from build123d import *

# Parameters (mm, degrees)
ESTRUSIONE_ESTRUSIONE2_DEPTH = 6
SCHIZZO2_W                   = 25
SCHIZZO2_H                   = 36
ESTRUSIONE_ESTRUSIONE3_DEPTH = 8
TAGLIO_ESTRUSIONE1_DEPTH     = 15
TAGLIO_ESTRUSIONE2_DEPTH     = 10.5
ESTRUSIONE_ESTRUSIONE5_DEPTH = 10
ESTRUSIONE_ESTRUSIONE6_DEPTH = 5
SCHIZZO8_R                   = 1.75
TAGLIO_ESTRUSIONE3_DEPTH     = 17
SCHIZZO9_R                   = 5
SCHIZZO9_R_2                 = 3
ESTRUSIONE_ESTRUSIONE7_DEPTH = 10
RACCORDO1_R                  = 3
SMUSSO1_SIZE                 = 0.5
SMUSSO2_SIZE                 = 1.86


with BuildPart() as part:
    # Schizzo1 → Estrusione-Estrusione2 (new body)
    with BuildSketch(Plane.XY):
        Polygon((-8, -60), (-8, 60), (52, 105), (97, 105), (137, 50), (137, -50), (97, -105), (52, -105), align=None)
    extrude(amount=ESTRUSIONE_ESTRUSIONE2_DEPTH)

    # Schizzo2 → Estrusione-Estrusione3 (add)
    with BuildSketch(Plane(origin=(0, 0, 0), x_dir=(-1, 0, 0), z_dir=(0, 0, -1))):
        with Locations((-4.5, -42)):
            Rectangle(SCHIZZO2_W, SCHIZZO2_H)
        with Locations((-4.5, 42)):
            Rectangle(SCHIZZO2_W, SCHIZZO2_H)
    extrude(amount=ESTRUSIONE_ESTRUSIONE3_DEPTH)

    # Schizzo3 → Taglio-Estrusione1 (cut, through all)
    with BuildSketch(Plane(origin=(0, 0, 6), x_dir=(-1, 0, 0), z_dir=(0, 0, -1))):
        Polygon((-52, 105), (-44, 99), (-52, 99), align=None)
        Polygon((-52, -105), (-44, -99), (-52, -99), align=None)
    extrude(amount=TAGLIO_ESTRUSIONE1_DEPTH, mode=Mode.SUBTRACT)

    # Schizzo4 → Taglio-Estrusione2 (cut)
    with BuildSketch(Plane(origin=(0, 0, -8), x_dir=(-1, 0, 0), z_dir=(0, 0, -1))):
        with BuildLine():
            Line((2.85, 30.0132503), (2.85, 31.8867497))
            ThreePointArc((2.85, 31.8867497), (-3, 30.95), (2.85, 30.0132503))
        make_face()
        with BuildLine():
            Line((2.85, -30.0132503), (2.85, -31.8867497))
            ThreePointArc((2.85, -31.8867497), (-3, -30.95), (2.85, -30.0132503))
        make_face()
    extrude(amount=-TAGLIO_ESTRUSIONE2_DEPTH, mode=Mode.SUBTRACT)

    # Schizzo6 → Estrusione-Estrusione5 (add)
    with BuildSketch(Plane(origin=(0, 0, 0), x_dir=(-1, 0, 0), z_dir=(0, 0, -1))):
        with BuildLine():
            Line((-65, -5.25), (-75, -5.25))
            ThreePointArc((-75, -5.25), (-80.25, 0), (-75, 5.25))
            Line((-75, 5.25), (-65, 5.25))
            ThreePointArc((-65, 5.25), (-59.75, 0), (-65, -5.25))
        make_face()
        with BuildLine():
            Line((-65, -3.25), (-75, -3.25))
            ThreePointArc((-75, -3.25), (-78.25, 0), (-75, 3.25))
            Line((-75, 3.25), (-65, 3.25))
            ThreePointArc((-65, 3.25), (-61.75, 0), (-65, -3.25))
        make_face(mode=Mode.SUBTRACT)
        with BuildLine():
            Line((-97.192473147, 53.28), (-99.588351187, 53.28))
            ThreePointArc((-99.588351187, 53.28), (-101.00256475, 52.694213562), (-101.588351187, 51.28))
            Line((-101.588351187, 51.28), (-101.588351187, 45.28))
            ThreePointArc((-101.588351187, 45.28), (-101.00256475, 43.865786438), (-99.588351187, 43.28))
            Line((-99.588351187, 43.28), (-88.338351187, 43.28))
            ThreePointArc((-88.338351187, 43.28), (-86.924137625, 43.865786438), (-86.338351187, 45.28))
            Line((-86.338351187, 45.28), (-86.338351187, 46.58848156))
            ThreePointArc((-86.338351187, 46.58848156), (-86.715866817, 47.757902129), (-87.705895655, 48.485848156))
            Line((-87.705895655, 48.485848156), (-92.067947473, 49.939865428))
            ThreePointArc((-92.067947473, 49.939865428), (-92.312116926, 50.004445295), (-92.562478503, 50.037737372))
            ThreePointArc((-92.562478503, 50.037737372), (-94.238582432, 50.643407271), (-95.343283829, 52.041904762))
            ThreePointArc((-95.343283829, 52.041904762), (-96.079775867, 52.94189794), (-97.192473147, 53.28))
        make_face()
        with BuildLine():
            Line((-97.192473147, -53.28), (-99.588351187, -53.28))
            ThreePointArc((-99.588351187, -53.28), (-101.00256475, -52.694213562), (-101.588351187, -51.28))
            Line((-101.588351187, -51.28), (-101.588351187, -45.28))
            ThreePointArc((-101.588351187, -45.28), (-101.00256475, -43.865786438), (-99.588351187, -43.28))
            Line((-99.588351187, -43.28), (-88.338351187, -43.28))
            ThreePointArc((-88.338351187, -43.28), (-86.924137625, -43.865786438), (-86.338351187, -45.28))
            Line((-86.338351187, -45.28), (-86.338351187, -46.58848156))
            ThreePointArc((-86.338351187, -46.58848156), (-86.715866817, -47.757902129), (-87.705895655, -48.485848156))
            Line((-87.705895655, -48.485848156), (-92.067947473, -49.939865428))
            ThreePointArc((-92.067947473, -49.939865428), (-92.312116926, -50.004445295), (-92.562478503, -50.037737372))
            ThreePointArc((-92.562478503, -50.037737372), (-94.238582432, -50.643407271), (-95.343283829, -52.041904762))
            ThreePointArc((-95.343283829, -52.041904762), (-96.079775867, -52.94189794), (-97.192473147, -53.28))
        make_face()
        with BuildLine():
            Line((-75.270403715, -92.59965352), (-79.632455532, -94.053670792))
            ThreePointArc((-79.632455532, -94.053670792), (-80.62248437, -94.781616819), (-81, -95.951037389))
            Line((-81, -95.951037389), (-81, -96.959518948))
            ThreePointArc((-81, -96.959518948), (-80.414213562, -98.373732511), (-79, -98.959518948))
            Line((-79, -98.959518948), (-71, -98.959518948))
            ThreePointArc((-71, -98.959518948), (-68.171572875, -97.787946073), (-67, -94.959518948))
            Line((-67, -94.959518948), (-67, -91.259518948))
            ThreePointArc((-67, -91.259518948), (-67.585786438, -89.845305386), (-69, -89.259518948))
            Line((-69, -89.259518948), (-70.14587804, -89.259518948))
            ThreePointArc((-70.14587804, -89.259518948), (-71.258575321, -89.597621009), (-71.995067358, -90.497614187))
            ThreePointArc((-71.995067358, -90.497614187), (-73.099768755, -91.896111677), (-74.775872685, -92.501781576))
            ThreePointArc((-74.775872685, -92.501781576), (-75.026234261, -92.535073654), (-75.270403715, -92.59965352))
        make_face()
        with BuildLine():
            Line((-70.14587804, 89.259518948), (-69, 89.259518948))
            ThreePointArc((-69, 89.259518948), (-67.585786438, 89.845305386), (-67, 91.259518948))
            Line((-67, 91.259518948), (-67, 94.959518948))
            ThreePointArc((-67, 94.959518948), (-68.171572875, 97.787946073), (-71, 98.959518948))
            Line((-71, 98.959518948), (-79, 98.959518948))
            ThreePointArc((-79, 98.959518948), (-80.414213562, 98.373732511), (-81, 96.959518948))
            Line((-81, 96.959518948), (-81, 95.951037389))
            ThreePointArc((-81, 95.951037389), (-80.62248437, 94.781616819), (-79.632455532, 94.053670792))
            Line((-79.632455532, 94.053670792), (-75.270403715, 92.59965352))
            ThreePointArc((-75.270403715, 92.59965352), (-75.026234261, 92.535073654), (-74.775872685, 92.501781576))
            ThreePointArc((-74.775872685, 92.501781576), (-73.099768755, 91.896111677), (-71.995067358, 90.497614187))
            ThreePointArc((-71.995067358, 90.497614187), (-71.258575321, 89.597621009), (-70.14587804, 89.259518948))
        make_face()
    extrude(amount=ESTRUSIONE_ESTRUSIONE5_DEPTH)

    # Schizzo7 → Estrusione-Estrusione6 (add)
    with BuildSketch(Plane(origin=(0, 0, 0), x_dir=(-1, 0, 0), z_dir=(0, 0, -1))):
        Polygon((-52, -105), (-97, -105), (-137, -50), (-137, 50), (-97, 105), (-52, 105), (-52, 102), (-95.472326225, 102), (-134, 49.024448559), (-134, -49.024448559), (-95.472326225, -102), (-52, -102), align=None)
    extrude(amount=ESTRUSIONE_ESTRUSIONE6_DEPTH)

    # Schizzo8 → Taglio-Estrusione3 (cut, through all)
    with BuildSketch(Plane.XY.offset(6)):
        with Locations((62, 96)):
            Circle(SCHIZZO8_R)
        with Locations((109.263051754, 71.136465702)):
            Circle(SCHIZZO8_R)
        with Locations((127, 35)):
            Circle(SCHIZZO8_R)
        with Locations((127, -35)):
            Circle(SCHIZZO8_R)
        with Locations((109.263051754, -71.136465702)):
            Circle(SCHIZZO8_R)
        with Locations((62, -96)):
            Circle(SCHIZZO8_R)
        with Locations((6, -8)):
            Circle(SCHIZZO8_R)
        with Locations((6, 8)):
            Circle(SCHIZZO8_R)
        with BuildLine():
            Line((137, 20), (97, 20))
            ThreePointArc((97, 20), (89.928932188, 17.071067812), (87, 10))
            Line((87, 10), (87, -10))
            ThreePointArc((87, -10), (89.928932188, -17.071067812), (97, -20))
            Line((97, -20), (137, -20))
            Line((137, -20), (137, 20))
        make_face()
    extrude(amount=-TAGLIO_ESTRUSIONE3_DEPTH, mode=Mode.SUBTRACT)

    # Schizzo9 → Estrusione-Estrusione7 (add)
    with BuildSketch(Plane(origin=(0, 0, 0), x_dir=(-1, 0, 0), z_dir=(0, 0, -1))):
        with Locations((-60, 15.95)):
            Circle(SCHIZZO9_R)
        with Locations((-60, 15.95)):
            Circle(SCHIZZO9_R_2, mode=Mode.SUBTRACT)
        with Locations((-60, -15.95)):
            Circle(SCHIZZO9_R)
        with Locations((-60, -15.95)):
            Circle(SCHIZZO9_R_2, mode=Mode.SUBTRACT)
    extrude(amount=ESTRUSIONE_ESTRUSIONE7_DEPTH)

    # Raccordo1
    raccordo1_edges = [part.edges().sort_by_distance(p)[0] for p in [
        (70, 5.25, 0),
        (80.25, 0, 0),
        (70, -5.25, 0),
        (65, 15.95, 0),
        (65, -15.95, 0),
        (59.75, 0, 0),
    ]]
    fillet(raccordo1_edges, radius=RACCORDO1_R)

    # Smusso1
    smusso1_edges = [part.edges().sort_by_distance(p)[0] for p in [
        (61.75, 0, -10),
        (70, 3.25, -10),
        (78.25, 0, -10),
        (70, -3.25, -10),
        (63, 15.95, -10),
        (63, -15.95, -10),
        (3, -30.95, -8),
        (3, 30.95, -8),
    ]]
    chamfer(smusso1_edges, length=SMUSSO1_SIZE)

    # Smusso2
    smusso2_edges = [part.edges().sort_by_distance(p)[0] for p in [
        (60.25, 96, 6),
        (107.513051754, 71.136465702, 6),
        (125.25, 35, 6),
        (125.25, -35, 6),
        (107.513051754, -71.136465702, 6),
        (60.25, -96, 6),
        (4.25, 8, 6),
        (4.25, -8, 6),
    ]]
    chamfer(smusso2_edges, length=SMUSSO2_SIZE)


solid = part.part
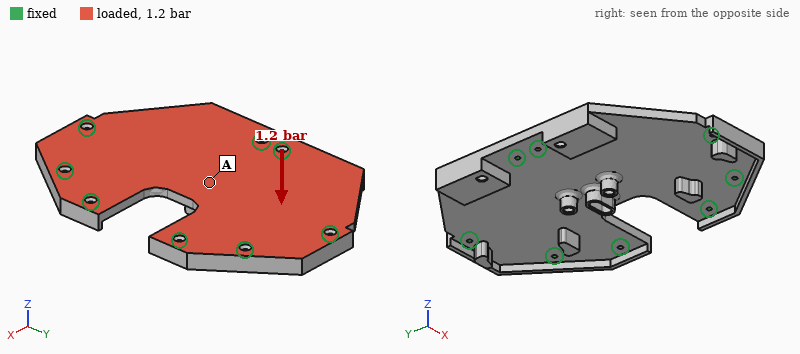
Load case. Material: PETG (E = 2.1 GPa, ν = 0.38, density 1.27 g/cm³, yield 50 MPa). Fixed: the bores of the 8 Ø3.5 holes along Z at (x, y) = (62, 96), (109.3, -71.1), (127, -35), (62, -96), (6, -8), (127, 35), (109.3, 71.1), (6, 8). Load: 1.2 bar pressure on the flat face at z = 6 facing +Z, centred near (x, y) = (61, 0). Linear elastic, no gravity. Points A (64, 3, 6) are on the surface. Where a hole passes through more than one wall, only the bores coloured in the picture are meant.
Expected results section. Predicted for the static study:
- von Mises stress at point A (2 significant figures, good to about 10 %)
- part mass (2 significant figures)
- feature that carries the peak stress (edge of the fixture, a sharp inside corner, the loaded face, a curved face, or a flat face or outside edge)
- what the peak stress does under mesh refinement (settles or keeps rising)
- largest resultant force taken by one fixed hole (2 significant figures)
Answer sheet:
6.6 MPa
210 g
edge of the fixture
keeps rising
510 N
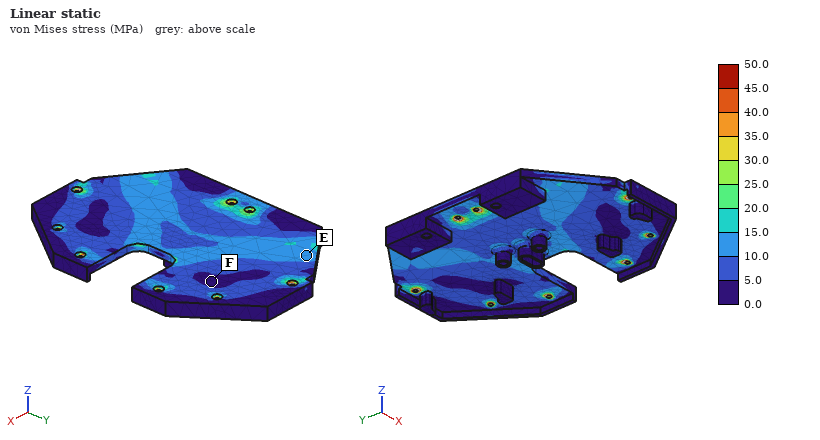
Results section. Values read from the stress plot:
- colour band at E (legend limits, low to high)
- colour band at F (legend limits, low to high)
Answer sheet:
10.0 to 15.0 MPa
0.0 to 5.0 MPa
